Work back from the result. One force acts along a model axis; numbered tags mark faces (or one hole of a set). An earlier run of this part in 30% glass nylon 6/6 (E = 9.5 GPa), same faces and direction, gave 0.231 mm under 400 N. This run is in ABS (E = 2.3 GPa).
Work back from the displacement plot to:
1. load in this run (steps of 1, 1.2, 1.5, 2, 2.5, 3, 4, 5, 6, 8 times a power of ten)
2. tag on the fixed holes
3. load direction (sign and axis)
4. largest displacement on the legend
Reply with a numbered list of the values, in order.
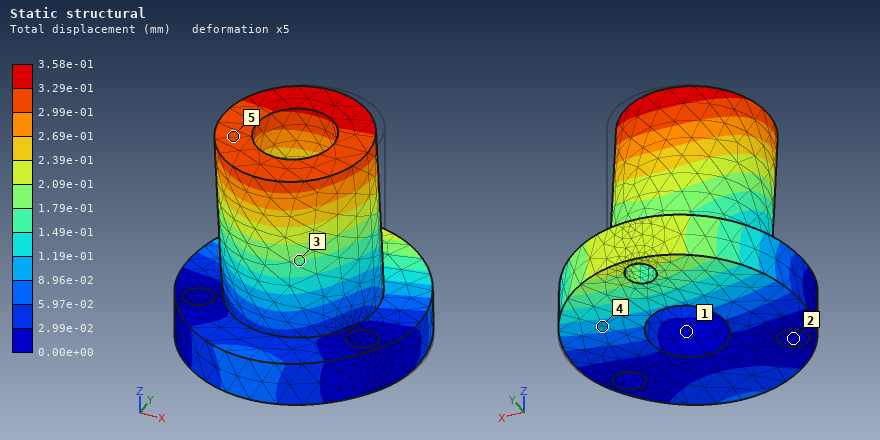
1. 150 N
2. 2
3. -Y
4. 3.58e-01 mm
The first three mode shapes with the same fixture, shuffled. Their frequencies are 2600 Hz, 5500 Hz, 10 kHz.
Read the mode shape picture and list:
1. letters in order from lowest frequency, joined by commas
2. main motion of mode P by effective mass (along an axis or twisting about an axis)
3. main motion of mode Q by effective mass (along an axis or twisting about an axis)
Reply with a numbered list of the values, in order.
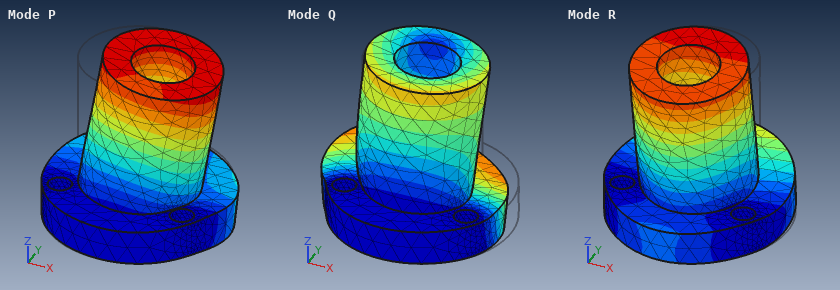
1. R, P, Q
2. along X
3. along X
